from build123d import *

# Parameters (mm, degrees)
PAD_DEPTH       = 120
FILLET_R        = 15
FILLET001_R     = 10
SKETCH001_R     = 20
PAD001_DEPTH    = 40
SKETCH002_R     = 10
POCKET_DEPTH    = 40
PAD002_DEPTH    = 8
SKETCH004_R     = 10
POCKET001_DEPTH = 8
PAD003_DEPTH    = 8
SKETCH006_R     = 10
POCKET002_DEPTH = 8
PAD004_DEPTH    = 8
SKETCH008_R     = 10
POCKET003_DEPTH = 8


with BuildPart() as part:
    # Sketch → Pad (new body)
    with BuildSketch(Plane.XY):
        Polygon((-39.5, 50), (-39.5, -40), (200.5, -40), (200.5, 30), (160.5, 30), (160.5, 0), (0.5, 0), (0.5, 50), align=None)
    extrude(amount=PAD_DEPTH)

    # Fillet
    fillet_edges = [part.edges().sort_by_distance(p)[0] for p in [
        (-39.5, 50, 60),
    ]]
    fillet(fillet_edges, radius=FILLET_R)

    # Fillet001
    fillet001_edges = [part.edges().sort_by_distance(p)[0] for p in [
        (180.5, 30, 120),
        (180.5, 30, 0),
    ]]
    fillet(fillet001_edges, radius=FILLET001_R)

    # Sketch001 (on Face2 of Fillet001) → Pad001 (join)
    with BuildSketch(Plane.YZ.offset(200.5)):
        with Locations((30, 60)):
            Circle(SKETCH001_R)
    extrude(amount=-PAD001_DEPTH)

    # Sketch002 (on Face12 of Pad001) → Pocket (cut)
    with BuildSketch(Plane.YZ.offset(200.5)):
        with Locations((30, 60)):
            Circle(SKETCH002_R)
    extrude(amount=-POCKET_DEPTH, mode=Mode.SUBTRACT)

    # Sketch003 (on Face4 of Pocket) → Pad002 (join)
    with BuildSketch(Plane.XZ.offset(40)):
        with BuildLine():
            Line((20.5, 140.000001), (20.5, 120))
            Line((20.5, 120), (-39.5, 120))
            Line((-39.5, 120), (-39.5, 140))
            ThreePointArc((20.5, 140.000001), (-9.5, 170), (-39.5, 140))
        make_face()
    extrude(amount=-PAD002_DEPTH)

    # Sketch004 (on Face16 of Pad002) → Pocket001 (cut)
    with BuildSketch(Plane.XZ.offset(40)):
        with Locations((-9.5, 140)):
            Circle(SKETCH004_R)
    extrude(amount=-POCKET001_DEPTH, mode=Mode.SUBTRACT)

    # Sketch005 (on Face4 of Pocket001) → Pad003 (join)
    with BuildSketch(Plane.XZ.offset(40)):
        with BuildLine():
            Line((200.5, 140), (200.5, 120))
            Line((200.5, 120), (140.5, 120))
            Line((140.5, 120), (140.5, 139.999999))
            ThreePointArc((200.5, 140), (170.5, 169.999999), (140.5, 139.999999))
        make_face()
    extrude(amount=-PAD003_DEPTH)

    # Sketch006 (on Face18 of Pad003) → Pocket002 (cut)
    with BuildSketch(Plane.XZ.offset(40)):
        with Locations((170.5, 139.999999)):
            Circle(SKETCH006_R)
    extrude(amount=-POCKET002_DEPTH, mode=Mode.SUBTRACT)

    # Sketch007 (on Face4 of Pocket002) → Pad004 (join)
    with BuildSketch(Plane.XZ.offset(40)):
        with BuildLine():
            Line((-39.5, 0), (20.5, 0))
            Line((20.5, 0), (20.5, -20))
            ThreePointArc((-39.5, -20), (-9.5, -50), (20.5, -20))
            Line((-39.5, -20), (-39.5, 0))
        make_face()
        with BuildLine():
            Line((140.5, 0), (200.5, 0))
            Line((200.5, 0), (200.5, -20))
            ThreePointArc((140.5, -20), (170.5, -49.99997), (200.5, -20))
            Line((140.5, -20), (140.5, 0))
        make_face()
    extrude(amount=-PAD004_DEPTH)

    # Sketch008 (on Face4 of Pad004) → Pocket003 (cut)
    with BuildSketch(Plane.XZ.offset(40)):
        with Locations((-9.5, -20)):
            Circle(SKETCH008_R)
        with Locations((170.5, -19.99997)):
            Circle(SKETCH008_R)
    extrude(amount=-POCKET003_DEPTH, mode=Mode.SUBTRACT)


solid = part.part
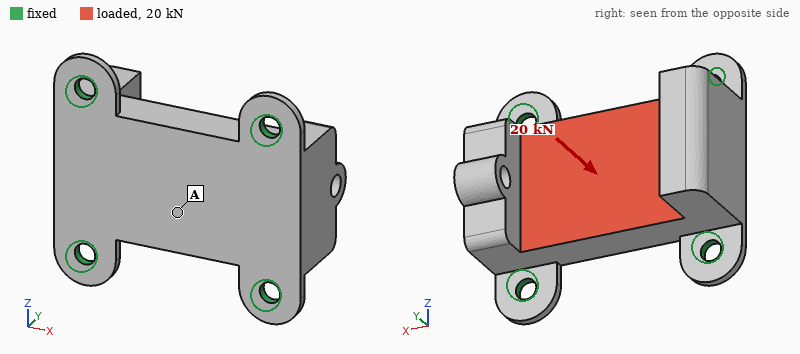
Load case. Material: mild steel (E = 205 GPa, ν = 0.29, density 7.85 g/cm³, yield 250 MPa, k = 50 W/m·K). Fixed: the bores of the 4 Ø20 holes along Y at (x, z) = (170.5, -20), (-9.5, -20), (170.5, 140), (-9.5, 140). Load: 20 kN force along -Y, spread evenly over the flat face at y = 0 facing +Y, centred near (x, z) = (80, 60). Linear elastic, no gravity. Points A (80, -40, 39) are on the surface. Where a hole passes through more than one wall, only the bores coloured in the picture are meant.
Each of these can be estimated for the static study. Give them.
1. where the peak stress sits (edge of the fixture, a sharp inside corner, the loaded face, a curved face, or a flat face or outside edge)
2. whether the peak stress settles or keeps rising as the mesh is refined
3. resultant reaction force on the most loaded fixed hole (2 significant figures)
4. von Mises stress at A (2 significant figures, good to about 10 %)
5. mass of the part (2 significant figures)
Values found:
edge of the fixture
keeps rising
6.3 kN
10 MPa
13 kg
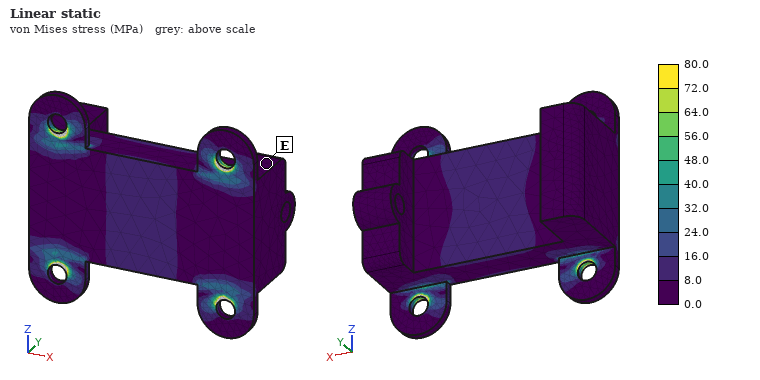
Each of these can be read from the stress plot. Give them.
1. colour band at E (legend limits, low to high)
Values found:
0.0 to 8.0 MPa
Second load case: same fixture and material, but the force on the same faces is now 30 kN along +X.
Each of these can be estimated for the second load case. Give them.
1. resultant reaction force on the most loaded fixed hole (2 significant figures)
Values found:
8.6 kN
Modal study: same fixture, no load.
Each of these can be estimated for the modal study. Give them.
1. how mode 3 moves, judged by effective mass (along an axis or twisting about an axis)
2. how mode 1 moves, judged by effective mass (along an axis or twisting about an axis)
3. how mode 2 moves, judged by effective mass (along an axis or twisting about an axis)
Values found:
along Z
along Y
along X
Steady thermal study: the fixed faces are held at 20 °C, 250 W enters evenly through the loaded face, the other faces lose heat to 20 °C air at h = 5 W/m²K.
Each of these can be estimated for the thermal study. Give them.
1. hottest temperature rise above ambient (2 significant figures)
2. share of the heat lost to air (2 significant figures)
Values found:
84 K
12 %
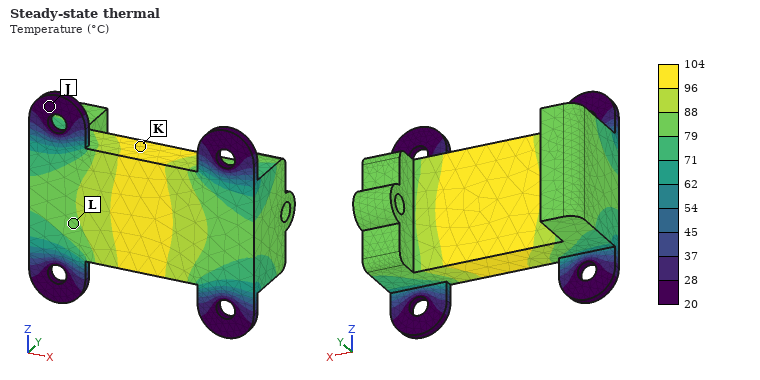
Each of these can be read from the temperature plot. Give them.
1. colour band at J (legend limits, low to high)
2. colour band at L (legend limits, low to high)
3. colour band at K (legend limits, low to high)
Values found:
20 to 28 °C
79 to 88 °C
96 to 104 °C
